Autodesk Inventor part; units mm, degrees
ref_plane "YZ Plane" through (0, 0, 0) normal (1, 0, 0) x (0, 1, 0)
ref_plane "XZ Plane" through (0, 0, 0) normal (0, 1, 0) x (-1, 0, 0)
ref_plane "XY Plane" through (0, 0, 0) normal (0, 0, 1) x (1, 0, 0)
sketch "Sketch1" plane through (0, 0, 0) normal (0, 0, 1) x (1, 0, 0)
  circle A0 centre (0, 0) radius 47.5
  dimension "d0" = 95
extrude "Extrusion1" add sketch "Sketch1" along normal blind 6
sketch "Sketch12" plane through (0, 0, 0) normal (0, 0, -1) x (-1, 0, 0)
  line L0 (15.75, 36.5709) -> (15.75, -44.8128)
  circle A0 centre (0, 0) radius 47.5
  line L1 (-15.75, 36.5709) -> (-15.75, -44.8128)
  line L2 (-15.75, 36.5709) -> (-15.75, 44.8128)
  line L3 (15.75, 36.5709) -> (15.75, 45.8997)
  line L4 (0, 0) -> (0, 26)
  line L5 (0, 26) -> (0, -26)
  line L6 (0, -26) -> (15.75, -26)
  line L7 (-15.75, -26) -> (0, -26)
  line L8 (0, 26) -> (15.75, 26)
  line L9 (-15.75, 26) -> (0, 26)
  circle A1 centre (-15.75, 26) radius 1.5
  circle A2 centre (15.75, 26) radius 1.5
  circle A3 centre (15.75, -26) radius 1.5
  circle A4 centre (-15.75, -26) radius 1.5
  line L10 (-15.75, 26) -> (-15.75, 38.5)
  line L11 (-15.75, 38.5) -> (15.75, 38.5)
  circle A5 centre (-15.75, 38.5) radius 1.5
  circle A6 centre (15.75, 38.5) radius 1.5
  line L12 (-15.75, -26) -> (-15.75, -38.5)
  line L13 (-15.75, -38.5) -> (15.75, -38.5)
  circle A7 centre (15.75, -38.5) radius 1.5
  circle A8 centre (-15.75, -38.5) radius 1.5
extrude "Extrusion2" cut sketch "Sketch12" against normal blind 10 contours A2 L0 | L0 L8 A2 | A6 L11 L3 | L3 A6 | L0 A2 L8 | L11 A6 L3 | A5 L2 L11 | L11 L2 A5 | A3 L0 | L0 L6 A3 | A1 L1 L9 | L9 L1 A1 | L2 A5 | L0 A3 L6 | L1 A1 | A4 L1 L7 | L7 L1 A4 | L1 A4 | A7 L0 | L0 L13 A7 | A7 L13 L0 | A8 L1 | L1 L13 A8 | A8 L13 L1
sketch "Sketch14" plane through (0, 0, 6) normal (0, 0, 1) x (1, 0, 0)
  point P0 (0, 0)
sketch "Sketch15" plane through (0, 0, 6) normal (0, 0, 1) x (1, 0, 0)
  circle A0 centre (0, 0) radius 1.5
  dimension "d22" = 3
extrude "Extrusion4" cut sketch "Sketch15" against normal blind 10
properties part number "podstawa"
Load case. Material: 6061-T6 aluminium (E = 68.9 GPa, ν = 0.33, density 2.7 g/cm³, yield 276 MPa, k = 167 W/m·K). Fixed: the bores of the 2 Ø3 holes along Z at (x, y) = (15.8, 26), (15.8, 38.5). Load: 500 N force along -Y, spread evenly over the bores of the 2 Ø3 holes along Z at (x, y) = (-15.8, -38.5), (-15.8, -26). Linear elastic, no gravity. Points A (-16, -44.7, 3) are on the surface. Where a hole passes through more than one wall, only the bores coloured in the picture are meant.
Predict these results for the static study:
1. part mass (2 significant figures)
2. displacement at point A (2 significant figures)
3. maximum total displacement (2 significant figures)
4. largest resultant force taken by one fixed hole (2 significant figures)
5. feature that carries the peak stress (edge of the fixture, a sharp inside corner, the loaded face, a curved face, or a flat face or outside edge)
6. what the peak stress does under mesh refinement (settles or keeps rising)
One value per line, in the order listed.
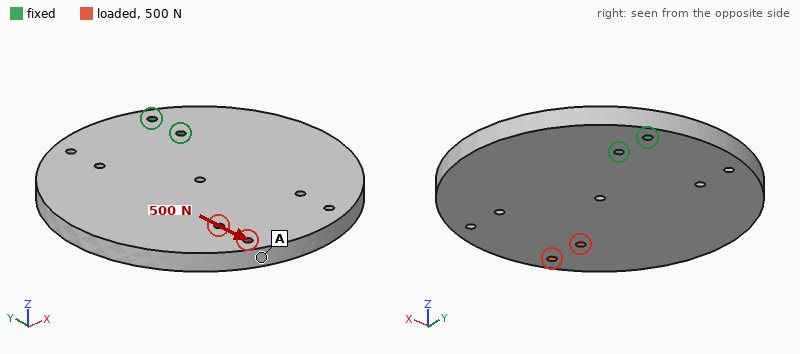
110 g
30 µm
30 µm
1.1 kN
edge of the fixture
keeps rising
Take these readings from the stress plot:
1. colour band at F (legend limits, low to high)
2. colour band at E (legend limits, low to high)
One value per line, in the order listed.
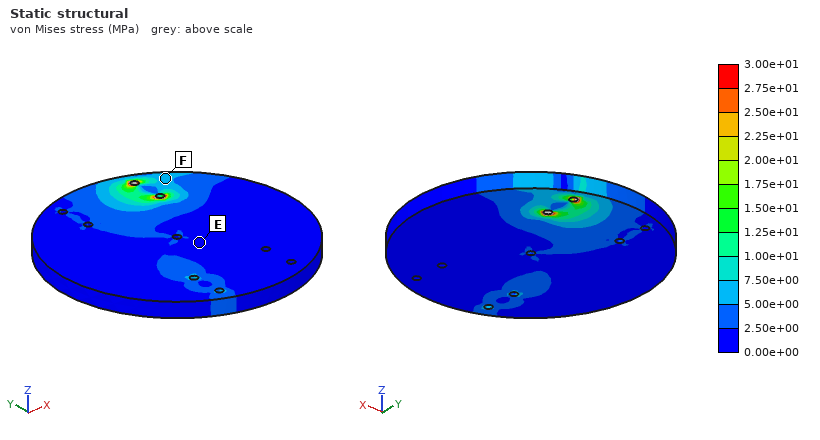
5.00e+00 to 7.50e+00 MPa
0.00e+00 to 2.50e+00 MPa
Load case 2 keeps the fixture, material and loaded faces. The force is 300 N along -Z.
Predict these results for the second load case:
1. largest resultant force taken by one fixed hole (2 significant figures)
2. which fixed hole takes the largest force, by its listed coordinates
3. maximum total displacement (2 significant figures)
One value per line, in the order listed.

1.0 kN
(15.8, 26)
0.54 mm
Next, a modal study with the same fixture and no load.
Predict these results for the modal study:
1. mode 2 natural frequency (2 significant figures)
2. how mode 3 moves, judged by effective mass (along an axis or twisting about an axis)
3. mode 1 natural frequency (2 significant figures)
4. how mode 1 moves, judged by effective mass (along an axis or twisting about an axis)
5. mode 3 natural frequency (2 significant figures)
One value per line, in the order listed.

1200 Hz
along X
730 Hz
along Z
2100 Hz
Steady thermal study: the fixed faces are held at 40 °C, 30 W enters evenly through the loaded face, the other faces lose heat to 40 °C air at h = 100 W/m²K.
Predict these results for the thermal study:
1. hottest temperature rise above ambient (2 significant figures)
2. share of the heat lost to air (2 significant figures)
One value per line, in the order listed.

28 K
55 %
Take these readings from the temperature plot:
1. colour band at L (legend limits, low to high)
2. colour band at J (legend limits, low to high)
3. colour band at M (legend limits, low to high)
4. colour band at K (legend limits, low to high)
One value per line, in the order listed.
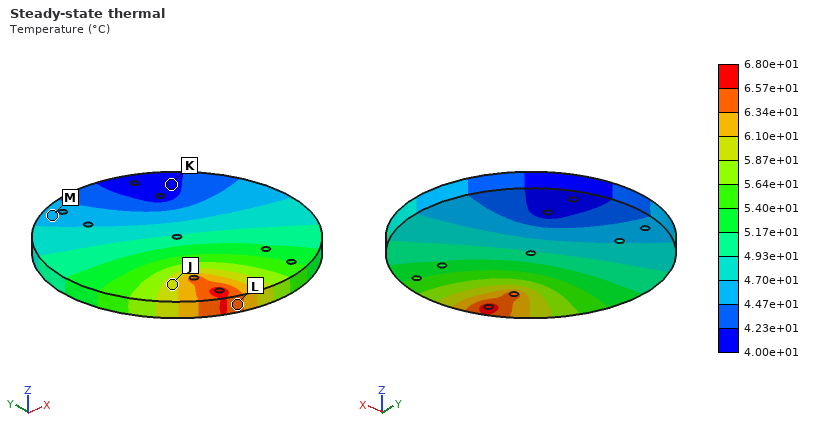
6.34e+01 to 6.57e+01 °C
5.87e+01 to 6.10e+01 °C
4.47e+01 to 4.70e+01 °C
4.00e+01 to 4.23e+01 °C
